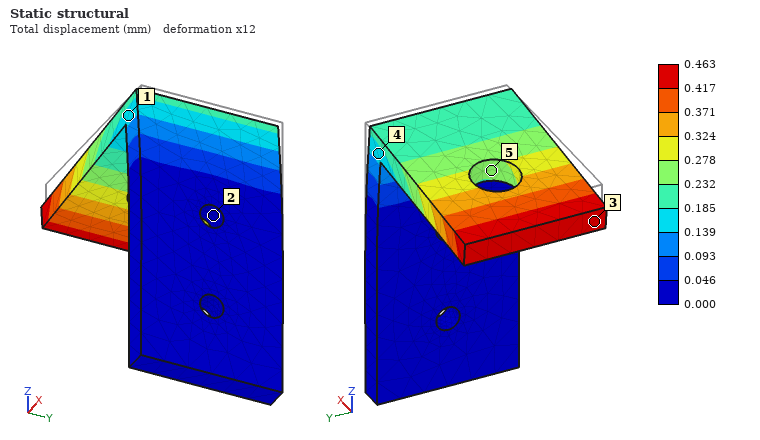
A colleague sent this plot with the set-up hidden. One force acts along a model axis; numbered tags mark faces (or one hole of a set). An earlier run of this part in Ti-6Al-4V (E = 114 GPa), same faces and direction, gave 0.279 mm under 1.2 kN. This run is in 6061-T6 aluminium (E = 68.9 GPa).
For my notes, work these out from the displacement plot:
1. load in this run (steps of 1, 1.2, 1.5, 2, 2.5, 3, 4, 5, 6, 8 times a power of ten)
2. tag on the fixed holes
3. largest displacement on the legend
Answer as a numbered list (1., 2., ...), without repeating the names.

1. 1.2 kN
2. 2
3. 0.463 mm
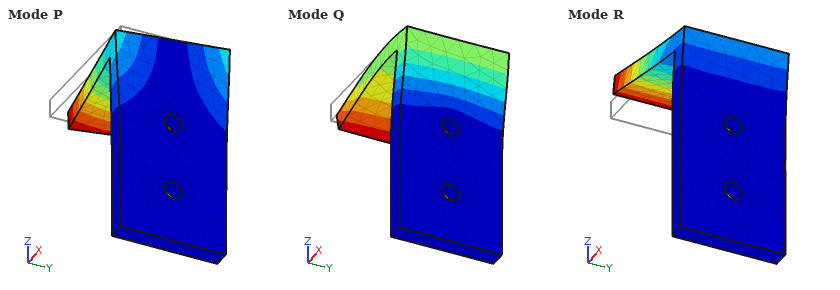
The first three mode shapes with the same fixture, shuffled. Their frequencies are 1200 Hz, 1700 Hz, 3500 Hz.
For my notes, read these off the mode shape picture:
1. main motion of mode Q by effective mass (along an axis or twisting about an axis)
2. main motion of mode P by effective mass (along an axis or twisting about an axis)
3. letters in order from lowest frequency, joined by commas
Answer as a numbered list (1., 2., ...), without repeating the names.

1. along X
2. along Y
3. R, P, Q
